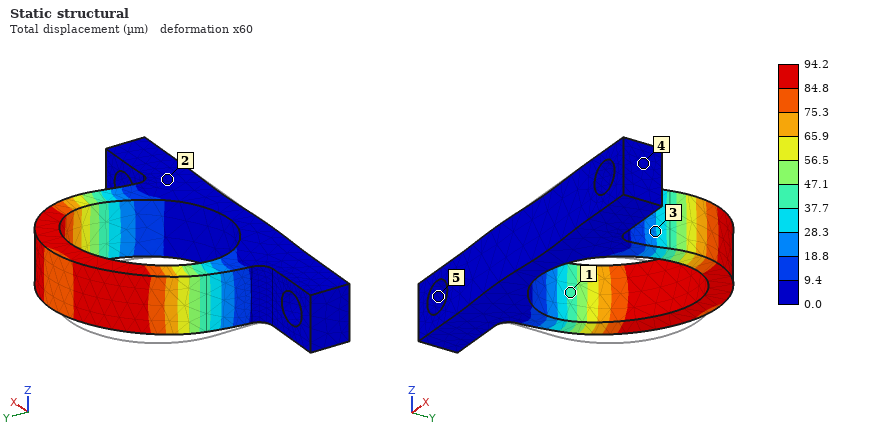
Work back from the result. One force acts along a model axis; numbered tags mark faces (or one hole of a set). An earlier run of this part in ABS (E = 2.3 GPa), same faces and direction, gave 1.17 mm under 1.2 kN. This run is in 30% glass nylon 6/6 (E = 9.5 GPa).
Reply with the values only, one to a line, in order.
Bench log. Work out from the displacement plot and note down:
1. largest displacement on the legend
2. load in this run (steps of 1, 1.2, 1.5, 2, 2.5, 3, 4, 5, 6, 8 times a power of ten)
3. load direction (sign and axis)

94.2 µm
400 N
+X
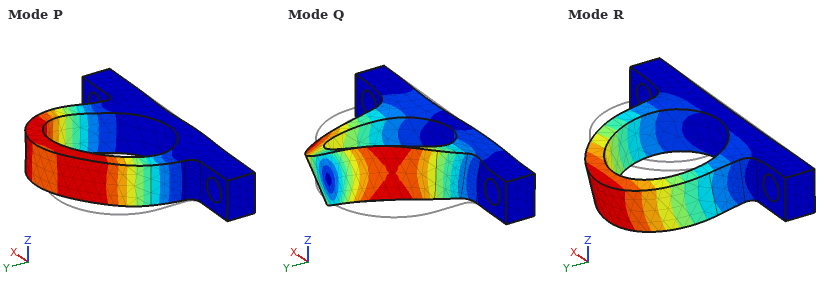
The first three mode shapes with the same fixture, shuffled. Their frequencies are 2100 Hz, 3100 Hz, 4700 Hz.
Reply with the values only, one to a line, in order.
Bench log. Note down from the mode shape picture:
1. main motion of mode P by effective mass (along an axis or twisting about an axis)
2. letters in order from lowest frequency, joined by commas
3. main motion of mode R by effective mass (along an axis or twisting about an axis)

along X
R, P, Q
along Z
